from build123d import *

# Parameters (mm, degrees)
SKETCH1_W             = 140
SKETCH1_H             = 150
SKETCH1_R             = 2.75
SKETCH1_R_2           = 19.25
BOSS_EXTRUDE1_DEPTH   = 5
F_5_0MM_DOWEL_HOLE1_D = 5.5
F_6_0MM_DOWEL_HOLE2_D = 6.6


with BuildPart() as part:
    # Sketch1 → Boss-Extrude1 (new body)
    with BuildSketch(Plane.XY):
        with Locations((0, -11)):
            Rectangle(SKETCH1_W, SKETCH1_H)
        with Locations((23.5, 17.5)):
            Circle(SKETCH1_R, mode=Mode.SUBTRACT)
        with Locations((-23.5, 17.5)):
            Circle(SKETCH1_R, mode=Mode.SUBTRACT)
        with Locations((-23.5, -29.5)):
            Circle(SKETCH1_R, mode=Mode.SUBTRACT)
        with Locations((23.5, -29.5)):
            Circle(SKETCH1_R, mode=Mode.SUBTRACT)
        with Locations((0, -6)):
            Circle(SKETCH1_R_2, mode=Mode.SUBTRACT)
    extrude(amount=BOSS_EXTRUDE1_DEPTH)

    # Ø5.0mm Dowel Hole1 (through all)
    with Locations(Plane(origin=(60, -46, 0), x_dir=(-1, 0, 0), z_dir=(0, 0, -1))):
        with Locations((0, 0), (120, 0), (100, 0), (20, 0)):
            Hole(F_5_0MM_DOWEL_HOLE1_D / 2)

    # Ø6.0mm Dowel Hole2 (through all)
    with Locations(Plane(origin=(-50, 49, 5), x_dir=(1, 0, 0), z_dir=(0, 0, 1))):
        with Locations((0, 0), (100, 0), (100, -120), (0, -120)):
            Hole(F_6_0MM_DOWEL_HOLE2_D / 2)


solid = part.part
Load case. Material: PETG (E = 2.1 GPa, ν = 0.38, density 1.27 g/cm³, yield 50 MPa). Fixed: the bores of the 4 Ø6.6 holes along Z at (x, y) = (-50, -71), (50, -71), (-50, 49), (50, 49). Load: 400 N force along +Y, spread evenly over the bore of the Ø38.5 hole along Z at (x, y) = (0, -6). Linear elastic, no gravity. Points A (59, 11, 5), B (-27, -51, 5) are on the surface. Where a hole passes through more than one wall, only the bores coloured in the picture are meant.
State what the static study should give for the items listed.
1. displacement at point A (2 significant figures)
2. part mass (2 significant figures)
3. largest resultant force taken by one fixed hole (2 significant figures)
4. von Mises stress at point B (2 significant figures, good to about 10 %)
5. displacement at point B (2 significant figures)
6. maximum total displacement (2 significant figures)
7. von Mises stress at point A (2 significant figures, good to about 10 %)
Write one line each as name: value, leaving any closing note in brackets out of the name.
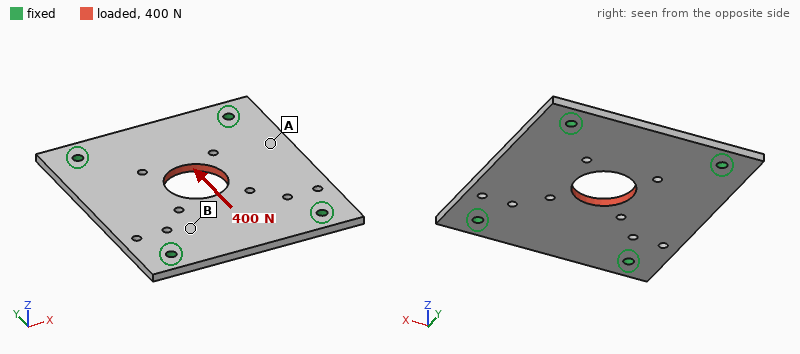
displacement at point A: 6.8 µm
part mass: 120 g
largest resultant force taken by one fixed hole: 110 N
von Mises stress at point B: 0.55 MPa
displacement at point B: 13 µm
maximum total displacement: 27 µm
von Mises stress at point A: 0.18 MPa
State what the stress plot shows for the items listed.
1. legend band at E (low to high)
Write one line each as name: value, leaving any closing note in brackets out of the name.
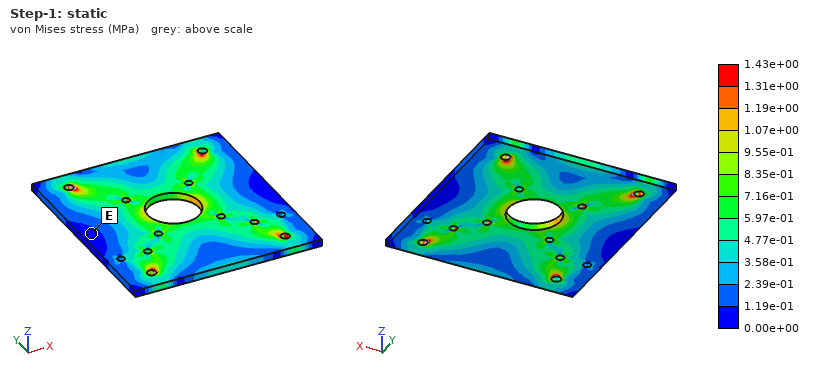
legend band at E: 0.00e+00 to 1.19e-01 MPa
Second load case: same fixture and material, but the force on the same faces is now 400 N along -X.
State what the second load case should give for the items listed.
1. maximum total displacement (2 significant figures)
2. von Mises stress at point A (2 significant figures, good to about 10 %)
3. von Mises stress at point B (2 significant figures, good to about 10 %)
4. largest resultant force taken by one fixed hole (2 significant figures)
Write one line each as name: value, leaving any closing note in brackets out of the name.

maximum total displacement: 32 µm
von Mises stress at point A: 0.32 MPa
von Mises stress at point B: 0.65 MPa
largest resultant force taken by one fixed hole: 120 N
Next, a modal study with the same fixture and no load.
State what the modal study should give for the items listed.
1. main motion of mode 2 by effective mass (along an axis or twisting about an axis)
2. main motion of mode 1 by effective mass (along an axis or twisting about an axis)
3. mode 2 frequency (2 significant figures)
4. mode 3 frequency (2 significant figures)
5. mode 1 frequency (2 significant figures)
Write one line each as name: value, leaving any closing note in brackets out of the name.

main motion of mode 2 by effective mass: twisting about Y
main motion of mode 1 by effective mass: along Z
mode 2 frequency: 510 Hz
mode 3 frequency: 590 Hz
mode 1 frequency: 380 Hz
